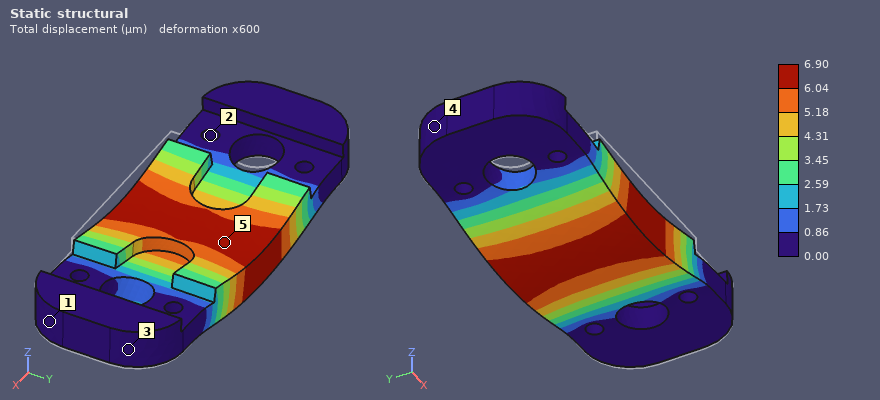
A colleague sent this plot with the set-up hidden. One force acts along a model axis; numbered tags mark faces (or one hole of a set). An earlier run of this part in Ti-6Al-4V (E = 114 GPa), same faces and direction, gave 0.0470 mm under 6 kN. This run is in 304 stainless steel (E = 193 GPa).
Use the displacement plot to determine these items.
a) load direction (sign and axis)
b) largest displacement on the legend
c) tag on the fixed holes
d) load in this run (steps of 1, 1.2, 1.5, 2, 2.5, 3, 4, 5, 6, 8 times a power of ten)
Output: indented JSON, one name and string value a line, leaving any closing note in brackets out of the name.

{
  "load direction": "-Z",
  "largest displacement on the legend": "6.90 µm",
  "tag on the fixed holes": "2",
  "load in this run": "1.5 kN"
}
